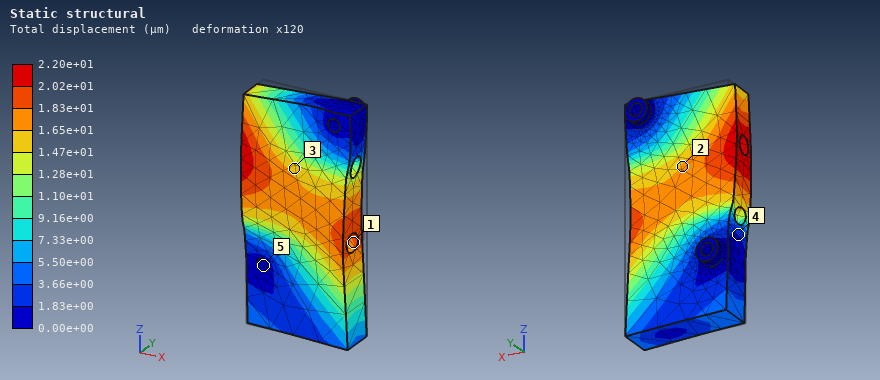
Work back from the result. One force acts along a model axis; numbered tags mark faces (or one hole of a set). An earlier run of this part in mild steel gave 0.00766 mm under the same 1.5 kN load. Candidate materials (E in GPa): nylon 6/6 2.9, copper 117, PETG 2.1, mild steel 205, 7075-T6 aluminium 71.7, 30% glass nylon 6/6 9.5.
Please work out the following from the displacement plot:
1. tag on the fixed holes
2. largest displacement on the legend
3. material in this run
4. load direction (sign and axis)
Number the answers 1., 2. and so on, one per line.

1. 5
2. 2.20e+01 µm
3. 7075-T6 aluminium
4. -Y
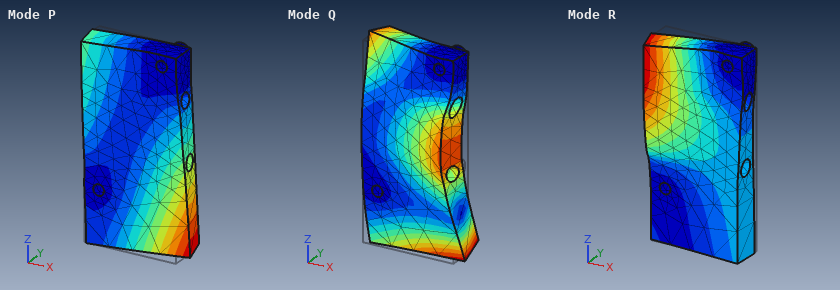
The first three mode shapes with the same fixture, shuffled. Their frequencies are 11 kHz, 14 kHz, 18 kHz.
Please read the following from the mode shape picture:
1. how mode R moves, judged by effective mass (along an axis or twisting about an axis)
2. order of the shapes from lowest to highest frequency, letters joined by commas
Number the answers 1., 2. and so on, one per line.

1. along Y
2. P, R, Q
